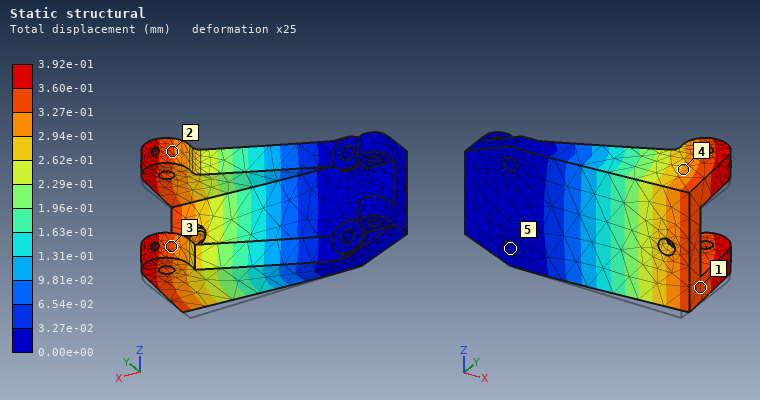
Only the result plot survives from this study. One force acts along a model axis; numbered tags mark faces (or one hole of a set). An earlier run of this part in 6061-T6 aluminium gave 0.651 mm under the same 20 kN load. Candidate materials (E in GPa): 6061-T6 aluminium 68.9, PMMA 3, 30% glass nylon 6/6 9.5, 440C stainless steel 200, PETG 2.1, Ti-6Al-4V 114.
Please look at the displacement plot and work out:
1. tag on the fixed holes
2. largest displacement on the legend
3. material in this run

5
3.92e-01 mm
Ti-6Al-4V
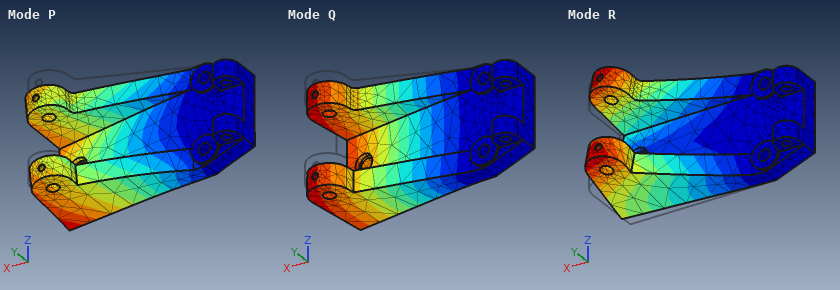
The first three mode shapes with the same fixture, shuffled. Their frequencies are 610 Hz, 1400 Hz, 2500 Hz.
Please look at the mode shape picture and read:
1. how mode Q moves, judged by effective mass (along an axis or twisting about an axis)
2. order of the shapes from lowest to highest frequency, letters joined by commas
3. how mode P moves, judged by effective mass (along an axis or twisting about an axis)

along Y
Q, R, P
along Z
